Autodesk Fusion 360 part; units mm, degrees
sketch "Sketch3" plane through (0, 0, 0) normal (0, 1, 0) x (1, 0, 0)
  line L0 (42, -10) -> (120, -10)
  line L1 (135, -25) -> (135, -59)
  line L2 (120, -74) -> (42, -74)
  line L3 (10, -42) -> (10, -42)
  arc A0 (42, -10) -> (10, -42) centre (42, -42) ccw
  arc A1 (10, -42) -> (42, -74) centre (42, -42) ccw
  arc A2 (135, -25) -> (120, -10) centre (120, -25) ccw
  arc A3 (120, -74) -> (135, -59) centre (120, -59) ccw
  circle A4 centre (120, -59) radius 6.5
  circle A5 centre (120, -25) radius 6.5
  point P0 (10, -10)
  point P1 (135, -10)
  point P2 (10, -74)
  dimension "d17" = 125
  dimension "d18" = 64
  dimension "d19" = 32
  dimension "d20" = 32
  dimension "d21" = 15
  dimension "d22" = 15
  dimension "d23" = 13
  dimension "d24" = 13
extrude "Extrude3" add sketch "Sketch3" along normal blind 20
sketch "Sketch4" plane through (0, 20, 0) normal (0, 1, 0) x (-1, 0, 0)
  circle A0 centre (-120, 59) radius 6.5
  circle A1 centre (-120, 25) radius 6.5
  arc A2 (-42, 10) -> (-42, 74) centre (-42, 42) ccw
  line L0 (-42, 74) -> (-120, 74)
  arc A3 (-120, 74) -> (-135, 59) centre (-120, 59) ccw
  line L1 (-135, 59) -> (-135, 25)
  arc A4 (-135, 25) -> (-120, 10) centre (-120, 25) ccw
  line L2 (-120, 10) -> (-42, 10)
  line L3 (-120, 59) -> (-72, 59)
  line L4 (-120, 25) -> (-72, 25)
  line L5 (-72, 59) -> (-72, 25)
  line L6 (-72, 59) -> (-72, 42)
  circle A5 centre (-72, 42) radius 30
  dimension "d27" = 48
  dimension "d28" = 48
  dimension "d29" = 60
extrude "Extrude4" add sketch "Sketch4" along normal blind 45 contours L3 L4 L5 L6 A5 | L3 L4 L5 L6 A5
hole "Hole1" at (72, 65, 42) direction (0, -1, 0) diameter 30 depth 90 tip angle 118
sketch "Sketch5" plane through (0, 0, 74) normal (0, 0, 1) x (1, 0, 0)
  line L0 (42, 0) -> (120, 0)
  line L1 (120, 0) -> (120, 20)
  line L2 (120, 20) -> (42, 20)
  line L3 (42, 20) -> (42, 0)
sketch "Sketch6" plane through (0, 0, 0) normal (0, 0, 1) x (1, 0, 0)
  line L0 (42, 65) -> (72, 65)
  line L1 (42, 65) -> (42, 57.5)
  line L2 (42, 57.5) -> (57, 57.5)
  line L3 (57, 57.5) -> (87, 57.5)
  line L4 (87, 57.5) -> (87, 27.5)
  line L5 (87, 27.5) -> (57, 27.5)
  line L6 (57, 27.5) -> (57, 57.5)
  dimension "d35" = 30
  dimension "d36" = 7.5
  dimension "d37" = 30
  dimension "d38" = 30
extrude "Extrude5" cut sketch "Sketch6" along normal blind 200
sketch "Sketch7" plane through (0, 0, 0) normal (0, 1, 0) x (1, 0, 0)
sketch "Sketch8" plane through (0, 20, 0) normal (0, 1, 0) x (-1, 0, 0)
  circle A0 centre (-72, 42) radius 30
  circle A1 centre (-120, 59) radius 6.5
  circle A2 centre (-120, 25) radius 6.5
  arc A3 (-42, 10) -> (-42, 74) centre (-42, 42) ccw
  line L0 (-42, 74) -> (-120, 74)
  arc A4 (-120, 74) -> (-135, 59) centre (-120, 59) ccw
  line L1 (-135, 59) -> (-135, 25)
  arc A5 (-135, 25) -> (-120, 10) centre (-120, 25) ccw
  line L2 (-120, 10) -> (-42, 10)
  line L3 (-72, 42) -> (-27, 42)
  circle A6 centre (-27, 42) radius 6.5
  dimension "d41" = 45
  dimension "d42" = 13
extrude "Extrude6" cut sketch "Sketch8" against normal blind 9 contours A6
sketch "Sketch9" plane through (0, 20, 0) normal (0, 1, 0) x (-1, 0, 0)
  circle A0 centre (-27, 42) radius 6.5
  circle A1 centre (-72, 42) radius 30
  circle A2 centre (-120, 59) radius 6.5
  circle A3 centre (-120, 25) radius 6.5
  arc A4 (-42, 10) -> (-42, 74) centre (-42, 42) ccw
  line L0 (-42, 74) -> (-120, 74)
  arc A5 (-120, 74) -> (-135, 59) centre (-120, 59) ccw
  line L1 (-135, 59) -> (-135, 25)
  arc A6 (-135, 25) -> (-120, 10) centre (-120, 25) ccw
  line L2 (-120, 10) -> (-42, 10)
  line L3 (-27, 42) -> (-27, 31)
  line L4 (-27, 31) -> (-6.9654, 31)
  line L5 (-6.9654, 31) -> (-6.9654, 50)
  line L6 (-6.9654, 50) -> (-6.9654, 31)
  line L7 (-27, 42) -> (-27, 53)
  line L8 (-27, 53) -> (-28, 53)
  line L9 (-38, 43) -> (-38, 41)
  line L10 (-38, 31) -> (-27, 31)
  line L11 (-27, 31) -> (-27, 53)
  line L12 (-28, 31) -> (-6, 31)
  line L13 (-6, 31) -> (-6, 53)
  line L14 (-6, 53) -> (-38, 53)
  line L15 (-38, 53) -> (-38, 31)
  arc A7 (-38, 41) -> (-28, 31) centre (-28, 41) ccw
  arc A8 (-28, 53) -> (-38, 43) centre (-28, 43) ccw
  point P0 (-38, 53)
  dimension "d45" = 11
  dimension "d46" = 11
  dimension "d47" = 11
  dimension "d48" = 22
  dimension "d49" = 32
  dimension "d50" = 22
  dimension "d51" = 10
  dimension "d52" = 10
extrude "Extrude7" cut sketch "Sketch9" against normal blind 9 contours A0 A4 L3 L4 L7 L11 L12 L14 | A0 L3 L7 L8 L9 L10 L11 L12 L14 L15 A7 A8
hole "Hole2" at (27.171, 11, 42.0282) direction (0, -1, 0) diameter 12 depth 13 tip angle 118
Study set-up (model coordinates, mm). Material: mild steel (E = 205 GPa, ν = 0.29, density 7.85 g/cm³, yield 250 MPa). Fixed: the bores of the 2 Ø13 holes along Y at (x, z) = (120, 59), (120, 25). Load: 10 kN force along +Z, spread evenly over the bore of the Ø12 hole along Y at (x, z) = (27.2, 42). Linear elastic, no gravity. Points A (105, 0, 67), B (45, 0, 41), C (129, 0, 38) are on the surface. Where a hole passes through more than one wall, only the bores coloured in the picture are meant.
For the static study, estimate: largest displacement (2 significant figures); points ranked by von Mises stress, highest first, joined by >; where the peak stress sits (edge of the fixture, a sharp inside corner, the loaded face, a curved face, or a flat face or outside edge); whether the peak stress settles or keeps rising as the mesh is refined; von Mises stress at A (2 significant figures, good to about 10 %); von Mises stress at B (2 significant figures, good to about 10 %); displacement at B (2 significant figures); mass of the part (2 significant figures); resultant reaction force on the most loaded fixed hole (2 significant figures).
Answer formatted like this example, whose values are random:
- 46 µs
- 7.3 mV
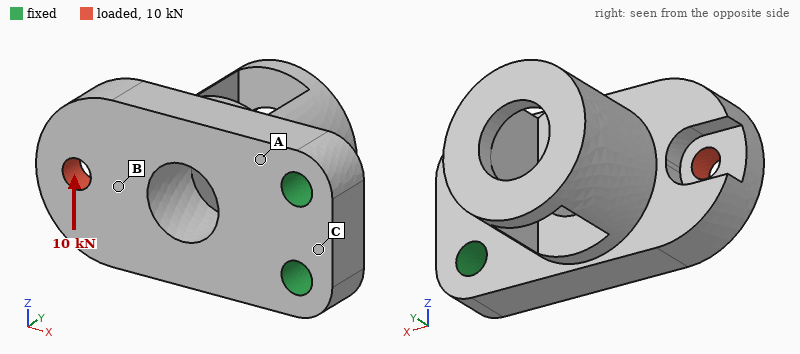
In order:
- 65 µm
- B > A > C
- edge of the fixture
- keeps rising
- 31 MPa
- 49 MPa
- 44 µm
- 1.5 kg
- 22 kN
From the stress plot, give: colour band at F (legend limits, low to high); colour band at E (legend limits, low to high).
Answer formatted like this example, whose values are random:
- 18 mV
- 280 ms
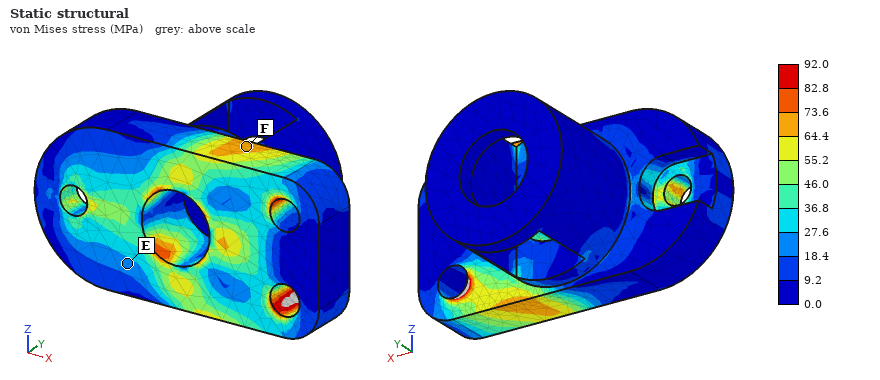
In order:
- 64.4 to 73.6 MPa
- 18.4 to 27.6 MPa
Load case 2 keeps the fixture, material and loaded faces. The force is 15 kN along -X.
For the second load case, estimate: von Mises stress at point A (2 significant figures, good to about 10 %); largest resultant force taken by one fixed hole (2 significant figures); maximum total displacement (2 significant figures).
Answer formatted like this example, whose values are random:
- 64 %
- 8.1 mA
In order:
- 33 MPa
- 7.5 kN
- 51 µm
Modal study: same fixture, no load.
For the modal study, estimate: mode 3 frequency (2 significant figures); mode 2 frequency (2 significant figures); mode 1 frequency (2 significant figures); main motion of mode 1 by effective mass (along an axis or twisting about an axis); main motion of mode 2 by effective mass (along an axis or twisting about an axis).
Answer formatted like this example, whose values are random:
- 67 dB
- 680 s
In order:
- 3800 Hz
- 3100 Hz
- 1400 Hz
- along Y
- along Z
